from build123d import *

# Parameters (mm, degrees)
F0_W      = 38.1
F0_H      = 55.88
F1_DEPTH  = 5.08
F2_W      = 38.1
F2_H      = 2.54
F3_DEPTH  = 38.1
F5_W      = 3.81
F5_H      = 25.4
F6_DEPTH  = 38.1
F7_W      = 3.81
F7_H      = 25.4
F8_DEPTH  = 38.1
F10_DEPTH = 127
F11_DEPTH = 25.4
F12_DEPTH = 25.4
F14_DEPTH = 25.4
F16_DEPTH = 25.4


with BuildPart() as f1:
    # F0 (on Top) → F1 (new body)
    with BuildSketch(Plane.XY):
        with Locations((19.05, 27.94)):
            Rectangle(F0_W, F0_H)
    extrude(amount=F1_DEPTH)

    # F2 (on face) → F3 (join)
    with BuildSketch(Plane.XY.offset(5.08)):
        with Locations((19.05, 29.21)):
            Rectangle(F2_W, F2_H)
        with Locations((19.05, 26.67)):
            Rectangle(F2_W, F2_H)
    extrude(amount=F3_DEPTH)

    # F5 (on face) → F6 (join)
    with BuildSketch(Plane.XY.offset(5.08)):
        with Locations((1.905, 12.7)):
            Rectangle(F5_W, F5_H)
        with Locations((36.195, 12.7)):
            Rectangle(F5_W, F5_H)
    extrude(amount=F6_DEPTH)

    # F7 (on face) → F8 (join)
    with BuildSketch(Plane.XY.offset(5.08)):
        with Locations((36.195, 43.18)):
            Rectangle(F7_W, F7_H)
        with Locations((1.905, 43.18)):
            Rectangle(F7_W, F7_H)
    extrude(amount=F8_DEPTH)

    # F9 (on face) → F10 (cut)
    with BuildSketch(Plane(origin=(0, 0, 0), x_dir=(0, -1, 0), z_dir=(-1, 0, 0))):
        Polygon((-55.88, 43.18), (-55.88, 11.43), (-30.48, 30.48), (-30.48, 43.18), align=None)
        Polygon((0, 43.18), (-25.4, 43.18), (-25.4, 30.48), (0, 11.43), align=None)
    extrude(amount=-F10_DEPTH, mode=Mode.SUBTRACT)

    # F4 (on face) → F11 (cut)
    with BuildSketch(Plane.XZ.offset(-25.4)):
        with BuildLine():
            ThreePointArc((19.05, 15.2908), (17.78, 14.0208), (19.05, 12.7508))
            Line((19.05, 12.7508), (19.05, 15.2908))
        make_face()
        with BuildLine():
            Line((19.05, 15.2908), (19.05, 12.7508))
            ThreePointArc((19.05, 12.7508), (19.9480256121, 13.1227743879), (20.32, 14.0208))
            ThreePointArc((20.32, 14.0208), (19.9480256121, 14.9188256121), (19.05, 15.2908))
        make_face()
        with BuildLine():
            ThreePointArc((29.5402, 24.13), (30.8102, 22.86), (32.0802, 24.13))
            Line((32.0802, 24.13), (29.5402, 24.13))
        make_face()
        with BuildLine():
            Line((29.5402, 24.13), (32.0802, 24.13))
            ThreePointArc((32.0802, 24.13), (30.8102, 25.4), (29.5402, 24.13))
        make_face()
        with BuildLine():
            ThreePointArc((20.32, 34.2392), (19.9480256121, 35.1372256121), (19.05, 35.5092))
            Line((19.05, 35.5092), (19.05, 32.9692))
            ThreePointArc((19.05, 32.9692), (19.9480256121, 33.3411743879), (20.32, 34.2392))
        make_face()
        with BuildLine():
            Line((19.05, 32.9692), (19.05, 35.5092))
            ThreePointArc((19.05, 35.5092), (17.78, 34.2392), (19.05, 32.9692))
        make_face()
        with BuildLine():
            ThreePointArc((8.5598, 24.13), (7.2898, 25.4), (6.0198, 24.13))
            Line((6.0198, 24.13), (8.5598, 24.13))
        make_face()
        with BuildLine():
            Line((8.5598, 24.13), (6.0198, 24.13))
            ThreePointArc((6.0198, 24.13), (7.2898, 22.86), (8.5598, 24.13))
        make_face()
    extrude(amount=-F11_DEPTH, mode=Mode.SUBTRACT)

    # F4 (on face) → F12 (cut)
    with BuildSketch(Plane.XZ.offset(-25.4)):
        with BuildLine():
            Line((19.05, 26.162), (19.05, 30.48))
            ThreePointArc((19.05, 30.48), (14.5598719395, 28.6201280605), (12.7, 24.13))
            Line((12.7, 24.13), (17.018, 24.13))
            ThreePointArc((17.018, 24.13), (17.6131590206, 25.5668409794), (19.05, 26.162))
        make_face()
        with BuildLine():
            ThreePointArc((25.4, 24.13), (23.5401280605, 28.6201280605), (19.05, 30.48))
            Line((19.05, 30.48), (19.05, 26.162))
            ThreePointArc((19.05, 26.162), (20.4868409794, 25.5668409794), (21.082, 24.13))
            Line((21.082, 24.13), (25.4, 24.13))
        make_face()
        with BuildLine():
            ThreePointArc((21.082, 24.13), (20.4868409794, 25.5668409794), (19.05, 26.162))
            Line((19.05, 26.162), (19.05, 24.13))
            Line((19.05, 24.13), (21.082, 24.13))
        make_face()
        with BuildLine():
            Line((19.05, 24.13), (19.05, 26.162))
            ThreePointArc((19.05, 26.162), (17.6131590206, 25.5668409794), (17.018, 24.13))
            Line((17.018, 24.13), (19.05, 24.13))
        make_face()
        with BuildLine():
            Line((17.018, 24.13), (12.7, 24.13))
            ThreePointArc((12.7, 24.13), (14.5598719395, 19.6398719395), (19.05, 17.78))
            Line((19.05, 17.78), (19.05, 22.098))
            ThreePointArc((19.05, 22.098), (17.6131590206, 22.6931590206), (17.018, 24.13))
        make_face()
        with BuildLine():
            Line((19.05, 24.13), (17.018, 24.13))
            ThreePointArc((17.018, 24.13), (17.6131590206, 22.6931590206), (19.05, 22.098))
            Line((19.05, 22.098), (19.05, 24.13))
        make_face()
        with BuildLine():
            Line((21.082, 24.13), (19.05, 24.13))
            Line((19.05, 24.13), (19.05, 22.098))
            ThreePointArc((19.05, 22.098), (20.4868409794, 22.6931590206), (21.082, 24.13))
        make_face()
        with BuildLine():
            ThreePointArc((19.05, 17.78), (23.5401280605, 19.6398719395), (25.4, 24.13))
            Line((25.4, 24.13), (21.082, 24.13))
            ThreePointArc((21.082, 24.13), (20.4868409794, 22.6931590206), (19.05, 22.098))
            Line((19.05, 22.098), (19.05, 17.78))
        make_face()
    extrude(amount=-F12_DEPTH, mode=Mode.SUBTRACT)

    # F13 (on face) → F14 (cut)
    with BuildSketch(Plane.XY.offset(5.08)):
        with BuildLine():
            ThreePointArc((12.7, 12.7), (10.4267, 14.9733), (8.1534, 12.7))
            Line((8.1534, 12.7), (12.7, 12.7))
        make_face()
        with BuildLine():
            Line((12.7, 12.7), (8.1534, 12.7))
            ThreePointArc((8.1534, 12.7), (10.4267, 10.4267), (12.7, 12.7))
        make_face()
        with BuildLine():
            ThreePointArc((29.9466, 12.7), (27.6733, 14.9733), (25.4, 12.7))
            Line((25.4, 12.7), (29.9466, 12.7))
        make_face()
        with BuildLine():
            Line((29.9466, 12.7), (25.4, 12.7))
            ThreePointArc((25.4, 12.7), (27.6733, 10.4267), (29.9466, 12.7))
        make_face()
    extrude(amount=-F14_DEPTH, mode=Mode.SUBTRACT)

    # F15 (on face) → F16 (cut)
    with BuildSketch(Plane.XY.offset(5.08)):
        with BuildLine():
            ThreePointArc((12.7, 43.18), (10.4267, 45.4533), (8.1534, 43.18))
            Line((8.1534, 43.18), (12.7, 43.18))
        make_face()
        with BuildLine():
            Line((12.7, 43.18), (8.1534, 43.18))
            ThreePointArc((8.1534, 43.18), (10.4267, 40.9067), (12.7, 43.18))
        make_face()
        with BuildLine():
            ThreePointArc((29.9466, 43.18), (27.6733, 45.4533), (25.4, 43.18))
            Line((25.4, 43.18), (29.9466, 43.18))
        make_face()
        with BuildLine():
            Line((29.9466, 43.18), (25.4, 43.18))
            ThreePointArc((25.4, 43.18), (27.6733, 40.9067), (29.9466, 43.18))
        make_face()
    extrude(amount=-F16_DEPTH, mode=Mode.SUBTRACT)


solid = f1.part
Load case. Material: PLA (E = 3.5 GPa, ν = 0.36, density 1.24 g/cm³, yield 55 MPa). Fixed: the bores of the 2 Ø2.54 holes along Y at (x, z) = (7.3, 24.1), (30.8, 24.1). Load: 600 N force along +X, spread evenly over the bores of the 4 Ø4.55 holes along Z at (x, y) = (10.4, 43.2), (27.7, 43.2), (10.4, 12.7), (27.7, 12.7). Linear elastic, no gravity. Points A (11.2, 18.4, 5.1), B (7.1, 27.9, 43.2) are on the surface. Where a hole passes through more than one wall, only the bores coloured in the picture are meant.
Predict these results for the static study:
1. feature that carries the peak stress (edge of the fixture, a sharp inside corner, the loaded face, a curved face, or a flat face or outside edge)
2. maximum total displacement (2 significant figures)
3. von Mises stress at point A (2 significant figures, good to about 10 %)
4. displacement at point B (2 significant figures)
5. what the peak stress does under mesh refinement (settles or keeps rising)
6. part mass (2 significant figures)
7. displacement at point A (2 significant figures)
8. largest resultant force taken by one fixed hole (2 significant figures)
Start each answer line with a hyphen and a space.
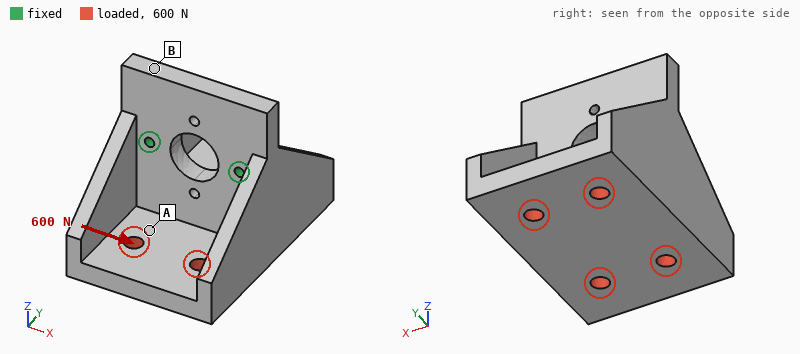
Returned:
- edge of the fixture
- 0.15 mm
- 4.0 MPa
- 0.037 mm
- keeps rising
- 29 g
- 0.12 mm
- 590 N
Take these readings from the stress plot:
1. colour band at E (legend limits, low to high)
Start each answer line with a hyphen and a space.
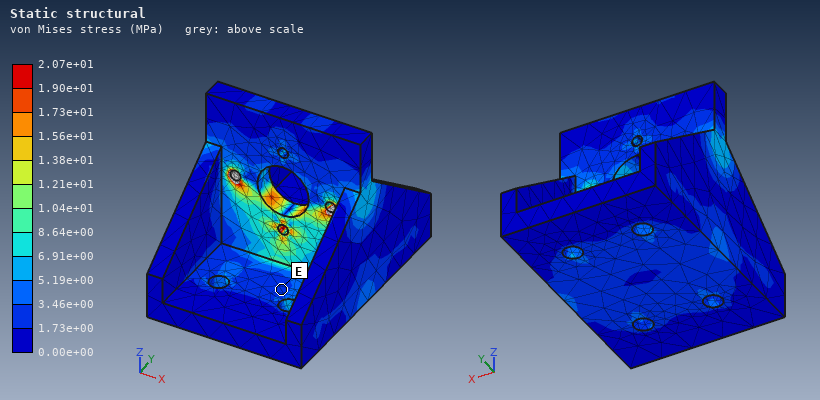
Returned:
- 1.73e+00 to 3.46e+00 MPa
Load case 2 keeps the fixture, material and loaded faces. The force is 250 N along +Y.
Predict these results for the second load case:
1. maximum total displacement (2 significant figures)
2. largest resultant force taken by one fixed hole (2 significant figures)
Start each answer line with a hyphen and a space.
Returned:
- 0.69 mm
- 130 N
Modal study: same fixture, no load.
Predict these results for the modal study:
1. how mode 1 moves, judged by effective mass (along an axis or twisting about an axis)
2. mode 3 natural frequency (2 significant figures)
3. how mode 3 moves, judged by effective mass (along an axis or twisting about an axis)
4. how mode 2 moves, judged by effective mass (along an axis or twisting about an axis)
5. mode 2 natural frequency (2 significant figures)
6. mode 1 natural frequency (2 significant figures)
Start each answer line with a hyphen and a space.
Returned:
- along Y
- 2500 Hz
- along X
- twisting about Z
- 1200 Hz
- 750 Hz
